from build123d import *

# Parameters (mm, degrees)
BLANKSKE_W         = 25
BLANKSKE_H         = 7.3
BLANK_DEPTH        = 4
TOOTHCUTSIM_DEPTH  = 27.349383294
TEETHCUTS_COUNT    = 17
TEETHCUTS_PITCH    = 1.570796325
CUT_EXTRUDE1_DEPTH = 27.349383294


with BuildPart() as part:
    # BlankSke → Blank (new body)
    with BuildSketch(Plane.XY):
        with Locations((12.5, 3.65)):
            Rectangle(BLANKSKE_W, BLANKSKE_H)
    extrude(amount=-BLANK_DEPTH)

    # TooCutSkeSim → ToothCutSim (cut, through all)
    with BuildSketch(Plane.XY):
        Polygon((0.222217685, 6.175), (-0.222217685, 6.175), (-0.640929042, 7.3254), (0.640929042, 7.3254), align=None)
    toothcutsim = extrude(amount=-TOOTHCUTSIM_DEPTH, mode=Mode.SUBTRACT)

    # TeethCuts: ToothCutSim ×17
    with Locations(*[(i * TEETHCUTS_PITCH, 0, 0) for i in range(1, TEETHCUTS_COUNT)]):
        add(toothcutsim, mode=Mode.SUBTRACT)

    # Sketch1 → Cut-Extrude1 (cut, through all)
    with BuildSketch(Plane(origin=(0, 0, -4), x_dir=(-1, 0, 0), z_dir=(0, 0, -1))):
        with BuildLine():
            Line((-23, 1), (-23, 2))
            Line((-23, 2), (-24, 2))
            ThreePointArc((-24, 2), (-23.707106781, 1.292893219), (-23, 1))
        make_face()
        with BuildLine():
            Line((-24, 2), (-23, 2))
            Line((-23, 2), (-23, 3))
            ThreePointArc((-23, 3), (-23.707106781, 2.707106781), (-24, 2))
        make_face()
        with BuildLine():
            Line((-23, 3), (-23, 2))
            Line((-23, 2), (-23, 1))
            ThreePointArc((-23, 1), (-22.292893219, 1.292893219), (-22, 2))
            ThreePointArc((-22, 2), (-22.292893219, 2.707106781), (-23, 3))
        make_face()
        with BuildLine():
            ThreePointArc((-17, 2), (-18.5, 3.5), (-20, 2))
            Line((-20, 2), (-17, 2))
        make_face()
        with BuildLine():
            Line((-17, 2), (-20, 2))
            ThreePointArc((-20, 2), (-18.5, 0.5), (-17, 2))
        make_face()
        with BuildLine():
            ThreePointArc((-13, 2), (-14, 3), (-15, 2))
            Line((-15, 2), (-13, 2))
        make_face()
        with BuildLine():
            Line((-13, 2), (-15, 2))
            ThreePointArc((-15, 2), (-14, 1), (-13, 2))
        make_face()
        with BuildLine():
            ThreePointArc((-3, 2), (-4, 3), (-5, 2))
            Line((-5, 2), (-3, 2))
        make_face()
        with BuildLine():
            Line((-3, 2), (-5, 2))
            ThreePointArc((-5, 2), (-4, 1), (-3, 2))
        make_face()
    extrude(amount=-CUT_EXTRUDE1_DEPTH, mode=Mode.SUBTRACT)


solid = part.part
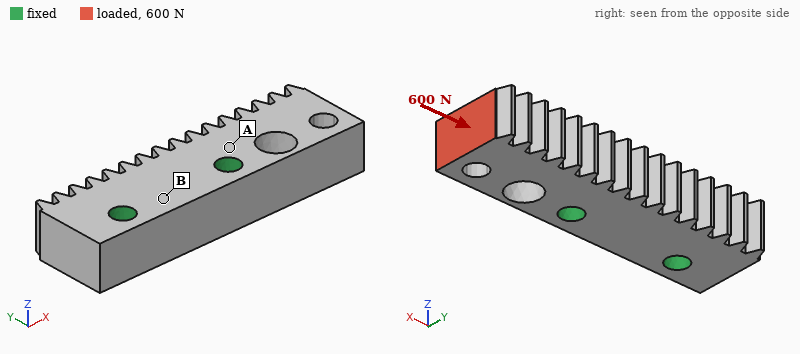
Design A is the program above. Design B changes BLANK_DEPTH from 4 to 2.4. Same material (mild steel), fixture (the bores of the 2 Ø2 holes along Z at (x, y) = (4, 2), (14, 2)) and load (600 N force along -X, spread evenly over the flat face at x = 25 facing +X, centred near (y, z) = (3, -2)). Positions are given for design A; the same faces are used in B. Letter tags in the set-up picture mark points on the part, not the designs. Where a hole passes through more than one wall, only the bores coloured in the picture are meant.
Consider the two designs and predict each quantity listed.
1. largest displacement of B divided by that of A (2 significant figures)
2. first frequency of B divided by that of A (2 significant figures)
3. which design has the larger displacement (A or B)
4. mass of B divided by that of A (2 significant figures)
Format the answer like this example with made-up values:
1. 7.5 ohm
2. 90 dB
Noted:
1. 1.7
2. 0.66
3. B
4. 0.60
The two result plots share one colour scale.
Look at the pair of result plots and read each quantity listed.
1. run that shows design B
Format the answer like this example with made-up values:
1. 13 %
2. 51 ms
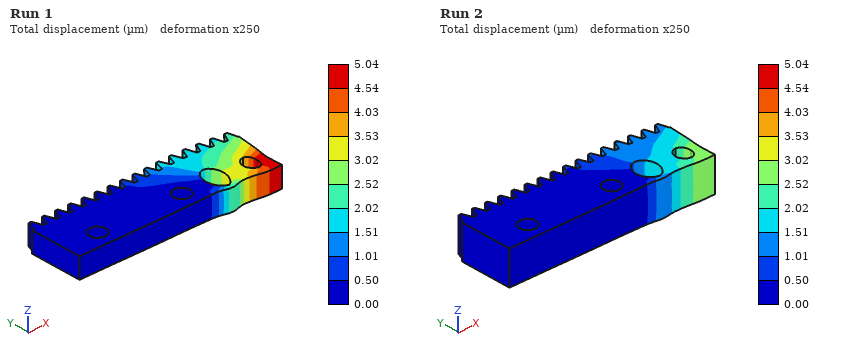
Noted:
1. Run 1
